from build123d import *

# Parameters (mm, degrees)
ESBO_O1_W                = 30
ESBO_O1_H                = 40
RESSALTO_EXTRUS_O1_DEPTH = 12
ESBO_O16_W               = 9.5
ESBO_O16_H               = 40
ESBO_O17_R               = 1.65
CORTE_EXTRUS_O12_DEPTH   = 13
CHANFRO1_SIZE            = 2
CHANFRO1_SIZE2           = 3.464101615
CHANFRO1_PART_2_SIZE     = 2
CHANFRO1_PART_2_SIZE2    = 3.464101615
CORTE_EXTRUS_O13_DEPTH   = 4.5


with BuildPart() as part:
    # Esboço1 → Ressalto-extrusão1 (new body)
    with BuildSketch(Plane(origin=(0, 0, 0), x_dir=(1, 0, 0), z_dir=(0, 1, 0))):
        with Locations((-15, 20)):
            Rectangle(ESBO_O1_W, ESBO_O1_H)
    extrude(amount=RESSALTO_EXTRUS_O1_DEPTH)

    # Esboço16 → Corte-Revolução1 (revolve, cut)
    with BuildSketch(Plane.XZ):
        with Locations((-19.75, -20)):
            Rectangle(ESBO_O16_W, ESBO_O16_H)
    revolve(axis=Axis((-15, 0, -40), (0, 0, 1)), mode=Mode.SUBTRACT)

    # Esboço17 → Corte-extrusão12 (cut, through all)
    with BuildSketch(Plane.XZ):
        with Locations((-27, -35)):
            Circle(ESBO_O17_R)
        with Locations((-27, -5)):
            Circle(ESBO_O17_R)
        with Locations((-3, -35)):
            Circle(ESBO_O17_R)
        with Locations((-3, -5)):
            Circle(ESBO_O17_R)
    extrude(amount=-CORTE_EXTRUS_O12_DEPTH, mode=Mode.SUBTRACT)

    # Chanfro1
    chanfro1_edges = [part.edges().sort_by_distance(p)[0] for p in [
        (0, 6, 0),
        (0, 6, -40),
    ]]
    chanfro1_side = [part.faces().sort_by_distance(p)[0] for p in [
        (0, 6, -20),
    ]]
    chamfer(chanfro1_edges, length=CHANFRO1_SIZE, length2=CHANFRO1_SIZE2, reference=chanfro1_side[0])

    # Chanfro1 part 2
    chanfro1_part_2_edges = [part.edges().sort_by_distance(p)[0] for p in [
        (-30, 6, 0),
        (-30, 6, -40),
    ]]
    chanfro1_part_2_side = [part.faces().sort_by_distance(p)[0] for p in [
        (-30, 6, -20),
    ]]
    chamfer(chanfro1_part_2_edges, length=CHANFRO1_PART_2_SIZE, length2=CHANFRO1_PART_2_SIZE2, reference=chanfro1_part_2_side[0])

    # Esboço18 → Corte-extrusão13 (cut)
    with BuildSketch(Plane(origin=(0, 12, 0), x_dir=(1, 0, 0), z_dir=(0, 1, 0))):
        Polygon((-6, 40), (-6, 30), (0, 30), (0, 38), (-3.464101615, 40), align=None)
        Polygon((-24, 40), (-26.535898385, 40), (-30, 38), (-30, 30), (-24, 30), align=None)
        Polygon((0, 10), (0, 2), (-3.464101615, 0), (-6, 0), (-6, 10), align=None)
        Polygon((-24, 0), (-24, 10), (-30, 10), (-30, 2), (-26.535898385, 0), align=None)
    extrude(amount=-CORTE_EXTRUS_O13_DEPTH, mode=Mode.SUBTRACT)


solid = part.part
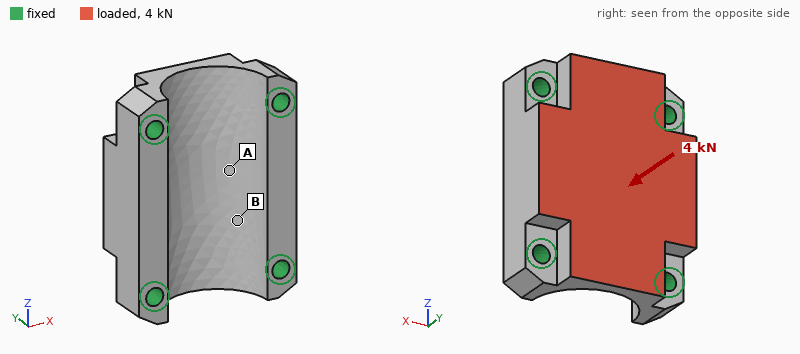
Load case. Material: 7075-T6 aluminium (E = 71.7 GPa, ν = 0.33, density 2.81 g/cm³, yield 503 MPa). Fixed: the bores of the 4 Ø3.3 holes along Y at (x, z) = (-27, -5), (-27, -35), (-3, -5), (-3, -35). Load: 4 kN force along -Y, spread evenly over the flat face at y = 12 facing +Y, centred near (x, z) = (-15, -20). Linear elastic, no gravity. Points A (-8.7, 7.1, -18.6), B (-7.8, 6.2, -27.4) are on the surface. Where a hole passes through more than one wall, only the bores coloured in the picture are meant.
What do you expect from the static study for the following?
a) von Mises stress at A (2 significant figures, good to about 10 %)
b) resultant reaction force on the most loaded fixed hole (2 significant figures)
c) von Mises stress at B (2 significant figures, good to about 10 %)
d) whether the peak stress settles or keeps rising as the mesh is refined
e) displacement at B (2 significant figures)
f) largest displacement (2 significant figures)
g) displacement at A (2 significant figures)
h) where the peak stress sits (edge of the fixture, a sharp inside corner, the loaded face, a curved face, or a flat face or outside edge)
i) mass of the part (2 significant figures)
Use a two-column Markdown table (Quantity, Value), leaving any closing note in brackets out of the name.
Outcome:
| Quantity | Value |
|---|---|
| von Mises stress at A | 12 MPa |
| resultant reaction force on the most loaded fixed hole | 1.2 kN |
| von Mises stress at B | 25 MPa |
| whether the peak stress settles or keeps rising as the mesh is refined | keeps rising |
| displacement at B | 6.1 µm |
| largest displacement | 12 µm |
| displacement at A | 8.4 µm |
| where the peak stress sits | edge of the fixture |
| mass of the part | 20 g |
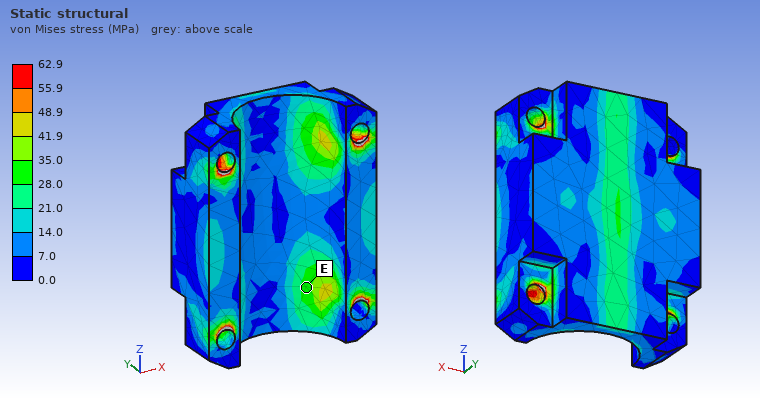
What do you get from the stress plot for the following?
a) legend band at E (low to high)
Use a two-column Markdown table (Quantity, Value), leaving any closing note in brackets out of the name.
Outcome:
| Quantity | Value |
|---|---|
| legend band at E | 28.0 to 35.0 MPa |
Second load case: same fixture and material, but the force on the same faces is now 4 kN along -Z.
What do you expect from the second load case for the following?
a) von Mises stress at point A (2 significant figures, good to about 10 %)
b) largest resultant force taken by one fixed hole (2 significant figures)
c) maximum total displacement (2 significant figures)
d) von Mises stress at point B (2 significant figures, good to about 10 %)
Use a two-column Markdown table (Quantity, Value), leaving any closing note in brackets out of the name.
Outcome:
| Quantity | Value |
|---|---|
| von Mises stress at point A | 20 MPa |
| largest resultant force taken by one fixed hole | 1.1 kN |
| maximum total displacement | 8.7 µm |
| von Mises stress at point B | 22 MPa |
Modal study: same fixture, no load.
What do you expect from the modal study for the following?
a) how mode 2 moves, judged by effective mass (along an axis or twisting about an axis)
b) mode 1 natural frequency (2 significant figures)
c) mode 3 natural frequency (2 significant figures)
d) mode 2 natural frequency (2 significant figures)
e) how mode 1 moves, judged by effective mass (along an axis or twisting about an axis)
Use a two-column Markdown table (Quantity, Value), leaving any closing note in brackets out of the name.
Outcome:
| Quantity | Value |
|---|---|
| how mode 2 moves, judged by effective mass | along Y |
| mode 1 natural frequency | 29 kHz |
| mode 3 natural frequency | 35 kHz |
| mode 2 natural frequency | 31 kHz |
| how mode 1 moves, judged by effective mass | along X |
